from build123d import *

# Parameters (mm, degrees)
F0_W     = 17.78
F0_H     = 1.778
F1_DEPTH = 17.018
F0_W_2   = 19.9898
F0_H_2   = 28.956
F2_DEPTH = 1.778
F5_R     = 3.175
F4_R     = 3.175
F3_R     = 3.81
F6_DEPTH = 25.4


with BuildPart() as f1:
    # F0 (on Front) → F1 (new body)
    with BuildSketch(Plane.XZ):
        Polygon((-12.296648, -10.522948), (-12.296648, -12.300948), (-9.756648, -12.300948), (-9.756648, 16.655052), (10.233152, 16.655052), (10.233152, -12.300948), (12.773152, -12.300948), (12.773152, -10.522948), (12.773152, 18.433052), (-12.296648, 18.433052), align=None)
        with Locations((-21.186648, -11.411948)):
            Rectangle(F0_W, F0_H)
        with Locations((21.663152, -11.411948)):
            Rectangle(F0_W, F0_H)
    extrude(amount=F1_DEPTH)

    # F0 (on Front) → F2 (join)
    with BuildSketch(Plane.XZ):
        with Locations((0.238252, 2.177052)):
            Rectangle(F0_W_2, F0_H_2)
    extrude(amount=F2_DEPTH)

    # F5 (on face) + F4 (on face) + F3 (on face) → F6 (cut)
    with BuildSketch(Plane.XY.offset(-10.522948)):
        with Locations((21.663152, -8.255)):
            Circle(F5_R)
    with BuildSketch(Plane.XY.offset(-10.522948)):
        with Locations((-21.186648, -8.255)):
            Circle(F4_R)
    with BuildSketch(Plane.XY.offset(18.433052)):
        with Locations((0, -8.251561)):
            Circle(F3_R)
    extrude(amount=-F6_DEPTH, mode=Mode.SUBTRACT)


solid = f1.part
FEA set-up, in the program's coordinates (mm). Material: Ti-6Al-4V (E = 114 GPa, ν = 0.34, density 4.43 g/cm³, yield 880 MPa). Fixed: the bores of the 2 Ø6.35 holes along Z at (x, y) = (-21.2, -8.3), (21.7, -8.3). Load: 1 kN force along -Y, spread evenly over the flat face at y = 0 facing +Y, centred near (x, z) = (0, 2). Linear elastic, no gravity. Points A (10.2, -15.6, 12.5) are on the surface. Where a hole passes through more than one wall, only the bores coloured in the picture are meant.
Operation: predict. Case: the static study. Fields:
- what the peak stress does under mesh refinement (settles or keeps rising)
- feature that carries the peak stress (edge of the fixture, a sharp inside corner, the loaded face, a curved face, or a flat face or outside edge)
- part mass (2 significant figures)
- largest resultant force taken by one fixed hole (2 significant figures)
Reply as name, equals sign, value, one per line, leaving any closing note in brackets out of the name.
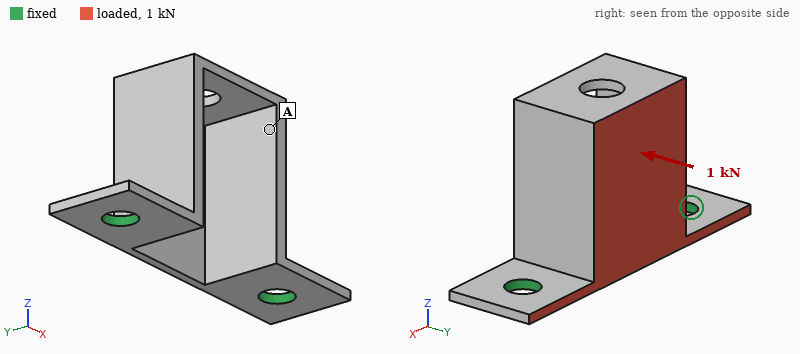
what the peak stress does under mesh refinement = keeps rising
feature that carries the peak stress = edge of the fixture
part mass = 23 g
largest resultant force taken by one fixed hole = 510 N
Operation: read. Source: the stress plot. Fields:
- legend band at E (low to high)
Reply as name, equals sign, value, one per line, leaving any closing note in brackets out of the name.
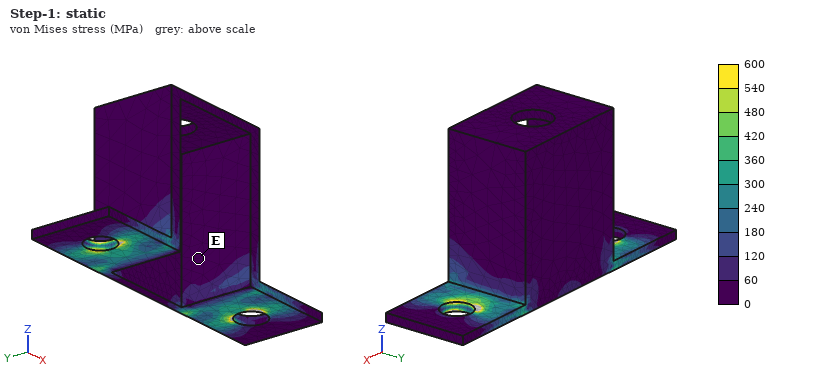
legend band at E = 0 to 60 MPa
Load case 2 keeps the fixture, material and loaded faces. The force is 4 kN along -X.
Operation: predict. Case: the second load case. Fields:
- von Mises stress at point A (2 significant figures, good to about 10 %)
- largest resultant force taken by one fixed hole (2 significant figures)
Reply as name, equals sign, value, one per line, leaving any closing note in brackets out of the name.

von Mises stress at point A = 87 MPa
largest resultant force taken by one fixed hole = 2.7 kN
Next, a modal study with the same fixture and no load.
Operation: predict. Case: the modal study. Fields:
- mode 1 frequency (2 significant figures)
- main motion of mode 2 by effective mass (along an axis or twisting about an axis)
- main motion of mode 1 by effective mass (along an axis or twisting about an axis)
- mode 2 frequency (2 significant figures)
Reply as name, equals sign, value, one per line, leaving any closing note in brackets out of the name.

mode 1 frequency = 1500 Hz
main motion of mode 2 by effective mass = along X
main motion of mode 1 by effective mass = along Y
mode 2 frequency = 2800 Hz
